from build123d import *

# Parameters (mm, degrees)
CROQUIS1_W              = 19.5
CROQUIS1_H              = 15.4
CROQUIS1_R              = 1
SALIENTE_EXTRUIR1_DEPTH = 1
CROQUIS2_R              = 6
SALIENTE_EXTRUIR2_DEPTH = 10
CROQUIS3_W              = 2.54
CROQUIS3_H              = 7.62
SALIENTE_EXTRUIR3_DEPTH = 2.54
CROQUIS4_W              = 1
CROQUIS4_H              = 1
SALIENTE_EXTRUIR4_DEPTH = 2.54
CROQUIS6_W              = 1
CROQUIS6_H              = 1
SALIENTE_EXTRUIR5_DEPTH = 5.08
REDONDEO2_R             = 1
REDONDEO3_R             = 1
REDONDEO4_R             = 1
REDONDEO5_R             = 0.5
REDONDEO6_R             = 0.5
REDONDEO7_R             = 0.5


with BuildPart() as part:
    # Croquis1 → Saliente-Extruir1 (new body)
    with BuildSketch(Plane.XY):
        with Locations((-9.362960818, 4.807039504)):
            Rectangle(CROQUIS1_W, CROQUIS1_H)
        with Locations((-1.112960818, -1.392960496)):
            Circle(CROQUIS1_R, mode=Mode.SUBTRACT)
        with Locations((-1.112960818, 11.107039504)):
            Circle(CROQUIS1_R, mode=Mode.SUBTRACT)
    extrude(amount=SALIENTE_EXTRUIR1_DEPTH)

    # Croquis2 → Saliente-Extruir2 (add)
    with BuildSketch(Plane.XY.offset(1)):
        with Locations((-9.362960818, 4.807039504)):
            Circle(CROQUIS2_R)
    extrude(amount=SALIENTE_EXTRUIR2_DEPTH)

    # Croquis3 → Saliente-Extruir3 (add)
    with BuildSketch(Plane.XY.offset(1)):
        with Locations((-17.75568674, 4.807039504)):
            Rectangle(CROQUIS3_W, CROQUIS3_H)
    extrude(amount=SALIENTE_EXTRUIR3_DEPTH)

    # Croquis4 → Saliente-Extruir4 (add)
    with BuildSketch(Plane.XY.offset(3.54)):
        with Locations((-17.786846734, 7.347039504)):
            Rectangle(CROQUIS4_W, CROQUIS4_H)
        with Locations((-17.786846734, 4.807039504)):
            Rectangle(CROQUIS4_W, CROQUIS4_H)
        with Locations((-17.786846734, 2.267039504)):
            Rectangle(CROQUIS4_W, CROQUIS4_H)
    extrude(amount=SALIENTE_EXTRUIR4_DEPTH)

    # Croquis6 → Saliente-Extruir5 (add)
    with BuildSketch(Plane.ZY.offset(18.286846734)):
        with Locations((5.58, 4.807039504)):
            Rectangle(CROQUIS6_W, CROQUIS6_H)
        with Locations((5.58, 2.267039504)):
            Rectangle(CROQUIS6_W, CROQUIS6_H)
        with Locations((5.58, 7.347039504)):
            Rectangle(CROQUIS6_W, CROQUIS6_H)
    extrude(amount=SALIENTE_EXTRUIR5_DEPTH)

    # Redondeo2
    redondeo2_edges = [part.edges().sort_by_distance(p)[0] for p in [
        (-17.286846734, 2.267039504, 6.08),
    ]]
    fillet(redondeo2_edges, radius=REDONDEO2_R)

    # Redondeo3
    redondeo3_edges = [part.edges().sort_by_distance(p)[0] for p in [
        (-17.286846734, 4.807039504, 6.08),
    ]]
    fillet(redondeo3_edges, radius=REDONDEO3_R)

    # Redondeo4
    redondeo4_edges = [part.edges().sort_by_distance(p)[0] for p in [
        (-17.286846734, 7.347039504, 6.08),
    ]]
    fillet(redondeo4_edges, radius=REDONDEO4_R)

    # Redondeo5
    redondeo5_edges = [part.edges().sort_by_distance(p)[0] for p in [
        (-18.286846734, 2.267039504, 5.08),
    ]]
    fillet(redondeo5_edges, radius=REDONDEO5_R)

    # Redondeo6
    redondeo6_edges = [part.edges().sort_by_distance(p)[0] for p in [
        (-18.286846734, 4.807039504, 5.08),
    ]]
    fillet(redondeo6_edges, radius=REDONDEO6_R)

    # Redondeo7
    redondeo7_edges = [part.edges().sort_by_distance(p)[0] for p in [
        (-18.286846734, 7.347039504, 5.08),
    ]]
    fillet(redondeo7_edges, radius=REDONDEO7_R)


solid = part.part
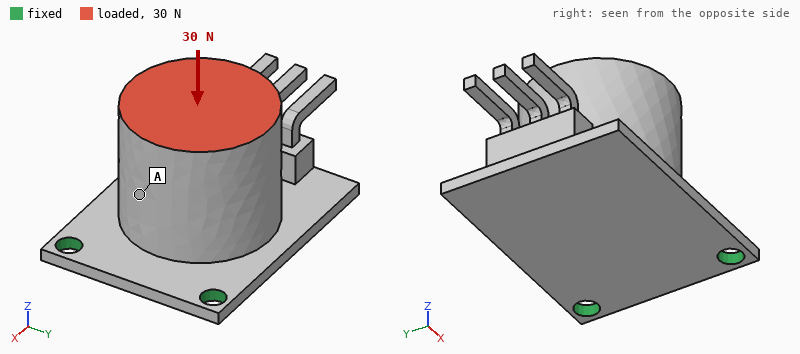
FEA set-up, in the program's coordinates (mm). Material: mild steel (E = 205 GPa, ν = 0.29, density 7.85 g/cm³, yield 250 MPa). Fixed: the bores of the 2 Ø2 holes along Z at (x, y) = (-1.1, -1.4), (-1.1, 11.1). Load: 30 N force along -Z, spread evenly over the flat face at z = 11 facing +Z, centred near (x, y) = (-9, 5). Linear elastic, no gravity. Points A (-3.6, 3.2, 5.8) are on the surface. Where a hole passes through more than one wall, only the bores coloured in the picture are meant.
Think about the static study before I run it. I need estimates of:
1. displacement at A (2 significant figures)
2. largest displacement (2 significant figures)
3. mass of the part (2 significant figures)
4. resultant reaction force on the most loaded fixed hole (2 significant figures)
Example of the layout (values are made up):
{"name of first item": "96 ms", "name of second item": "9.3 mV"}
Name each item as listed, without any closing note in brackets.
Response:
{"displacement at A": "13 µm", "largest displacement": "52 µm", "mass of the part": "12 g", "resultant reaction force on the most loaded fixed hole": "15 N"}
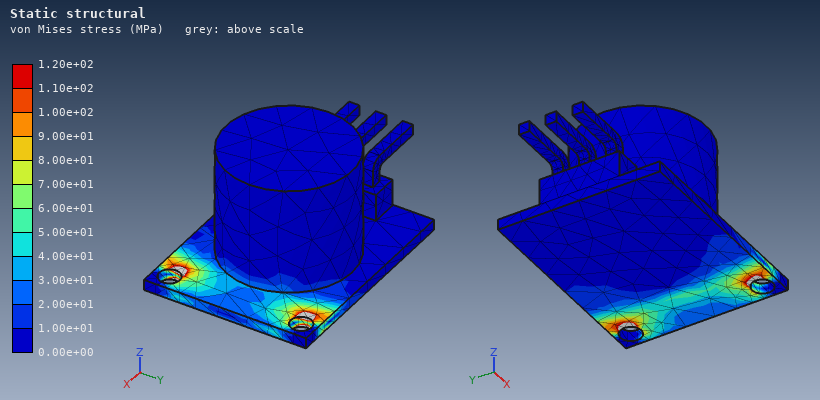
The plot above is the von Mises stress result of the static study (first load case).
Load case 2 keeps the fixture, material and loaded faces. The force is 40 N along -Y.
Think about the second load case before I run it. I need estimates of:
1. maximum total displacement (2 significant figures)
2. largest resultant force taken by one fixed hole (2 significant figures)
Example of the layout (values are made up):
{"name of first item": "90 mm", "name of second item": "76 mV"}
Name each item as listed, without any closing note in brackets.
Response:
{"maximum total displacement": "8.1 µm", "largest resultant force taken by one fixed hole": "51 N"}
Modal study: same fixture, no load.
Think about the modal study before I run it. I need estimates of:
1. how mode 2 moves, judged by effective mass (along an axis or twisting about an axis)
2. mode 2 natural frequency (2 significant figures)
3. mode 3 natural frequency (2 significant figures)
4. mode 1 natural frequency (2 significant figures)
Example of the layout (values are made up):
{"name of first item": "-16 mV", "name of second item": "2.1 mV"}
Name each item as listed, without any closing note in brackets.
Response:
{"how mode 2 moves, judged by effective mass": "along Y", "mode 2 natural frequency": "5800 Hz", "mode 3 natural frequency": "11 kHz", "mode 1 natural frequency": "1300 Hz"}
